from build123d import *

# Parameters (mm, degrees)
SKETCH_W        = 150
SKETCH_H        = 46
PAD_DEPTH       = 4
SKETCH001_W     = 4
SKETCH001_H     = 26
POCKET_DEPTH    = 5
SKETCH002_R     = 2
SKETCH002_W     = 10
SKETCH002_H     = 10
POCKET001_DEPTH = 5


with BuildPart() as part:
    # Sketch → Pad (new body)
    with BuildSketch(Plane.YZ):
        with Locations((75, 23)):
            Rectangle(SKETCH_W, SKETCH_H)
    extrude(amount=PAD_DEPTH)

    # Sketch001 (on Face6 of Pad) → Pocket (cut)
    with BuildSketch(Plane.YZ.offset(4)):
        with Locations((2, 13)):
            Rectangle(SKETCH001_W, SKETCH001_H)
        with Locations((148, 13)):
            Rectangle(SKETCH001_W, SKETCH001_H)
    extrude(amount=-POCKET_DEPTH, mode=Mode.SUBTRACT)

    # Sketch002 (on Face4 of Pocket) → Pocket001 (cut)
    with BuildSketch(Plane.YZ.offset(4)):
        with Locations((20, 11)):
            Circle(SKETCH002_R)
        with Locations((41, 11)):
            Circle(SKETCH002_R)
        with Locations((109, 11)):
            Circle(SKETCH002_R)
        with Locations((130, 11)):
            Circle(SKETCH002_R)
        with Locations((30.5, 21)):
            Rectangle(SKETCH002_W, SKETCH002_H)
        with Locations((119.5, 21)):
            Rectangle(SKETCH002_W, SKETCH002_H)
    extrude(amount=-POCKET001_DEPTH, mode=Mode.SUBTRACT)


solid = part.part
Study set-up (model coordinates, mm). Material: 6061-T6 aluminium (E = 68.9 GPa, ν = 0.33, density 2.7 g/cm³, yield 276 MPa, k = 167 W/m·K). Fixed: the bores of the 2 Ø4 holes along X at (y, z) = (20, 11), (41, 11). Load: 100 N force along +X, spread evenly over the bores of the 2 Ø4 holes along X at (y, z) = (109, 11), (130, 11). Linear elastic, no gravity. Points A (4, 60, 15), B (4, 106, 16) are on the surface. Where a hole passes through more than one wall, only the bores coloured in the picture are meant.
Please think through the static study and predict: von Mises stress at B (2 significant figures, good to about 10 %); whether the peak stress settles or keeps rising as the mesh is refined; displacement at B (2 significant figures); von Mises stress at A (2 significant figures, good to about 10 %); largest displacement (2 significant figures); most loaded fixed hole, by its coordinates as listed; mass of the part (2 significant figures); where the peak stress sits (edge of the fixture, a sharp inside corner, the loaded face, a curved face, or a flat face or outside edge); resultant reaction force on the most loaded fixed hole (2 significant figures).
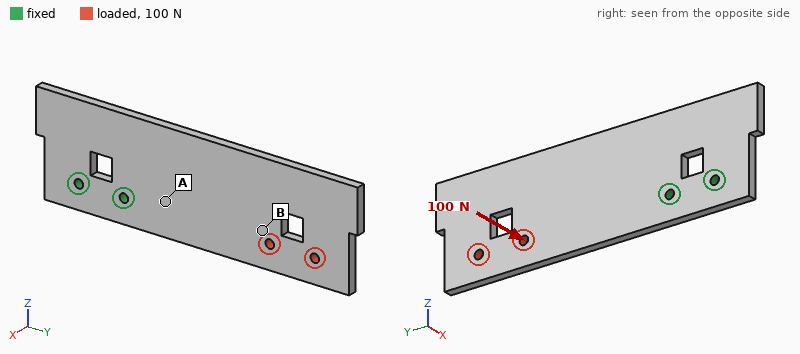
15 MPa
keeps rising
0.82 mm
47 MPa
1.7 mm
(41, 11)
70 g
edge of the fixture
250 N
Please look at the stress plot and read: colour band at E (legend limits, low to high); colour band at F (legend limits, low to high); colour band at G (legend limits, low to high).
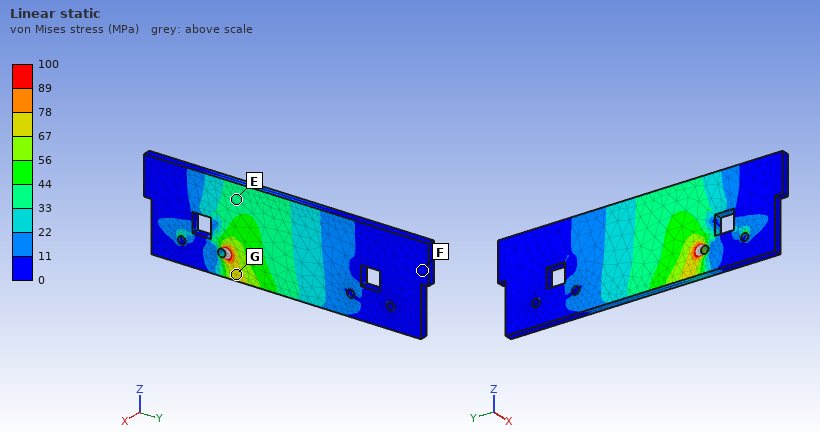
33 to 44 MPa
0 to 11 MPa
67 to 78 MPa
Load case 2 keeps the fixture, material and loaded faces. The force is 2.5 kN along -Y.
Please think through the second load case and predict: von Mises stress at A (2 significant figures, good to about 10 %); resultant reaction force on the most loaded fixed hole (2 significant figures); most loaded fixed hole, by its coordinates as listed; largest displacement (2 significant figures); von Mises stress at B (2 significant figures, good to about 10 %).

22 MPa
2.0 kN
(41, 11)
71 µm
28 MPa
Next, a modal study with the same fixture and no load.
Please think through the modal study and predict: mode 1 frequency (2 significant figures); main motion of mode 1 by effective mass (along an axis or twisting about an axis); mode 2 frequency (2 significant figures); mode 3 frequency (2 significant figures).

270 Hz
along X
1100 Hz
1600 Hz
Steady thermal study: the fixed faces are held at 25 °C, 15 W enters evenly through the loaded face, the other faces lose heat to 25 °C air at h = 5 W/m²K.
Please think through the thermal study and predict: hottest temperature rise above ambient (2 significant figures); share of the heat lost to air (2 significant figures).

46 K
10 %
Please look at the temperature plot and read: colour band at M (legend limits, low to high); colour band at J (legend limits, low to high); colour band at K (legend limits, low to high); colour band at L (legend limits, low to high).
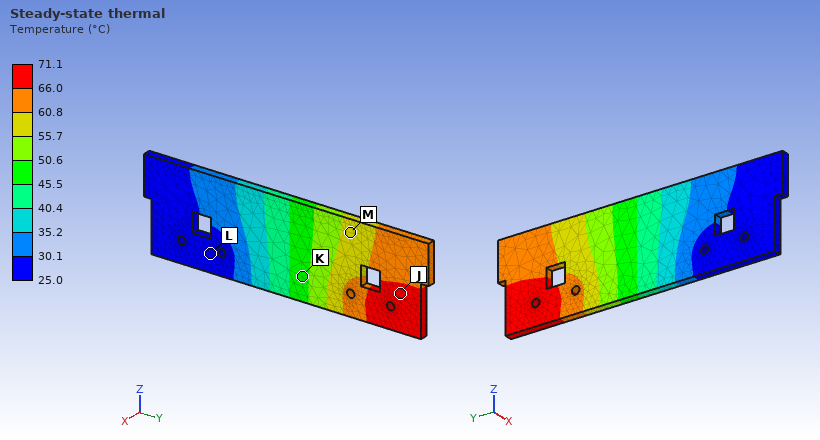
55.7 to 60.8 °C
66.0 to 71.1 °C
45.5 to 50.6 °C
25.0 to 30.1 °C
